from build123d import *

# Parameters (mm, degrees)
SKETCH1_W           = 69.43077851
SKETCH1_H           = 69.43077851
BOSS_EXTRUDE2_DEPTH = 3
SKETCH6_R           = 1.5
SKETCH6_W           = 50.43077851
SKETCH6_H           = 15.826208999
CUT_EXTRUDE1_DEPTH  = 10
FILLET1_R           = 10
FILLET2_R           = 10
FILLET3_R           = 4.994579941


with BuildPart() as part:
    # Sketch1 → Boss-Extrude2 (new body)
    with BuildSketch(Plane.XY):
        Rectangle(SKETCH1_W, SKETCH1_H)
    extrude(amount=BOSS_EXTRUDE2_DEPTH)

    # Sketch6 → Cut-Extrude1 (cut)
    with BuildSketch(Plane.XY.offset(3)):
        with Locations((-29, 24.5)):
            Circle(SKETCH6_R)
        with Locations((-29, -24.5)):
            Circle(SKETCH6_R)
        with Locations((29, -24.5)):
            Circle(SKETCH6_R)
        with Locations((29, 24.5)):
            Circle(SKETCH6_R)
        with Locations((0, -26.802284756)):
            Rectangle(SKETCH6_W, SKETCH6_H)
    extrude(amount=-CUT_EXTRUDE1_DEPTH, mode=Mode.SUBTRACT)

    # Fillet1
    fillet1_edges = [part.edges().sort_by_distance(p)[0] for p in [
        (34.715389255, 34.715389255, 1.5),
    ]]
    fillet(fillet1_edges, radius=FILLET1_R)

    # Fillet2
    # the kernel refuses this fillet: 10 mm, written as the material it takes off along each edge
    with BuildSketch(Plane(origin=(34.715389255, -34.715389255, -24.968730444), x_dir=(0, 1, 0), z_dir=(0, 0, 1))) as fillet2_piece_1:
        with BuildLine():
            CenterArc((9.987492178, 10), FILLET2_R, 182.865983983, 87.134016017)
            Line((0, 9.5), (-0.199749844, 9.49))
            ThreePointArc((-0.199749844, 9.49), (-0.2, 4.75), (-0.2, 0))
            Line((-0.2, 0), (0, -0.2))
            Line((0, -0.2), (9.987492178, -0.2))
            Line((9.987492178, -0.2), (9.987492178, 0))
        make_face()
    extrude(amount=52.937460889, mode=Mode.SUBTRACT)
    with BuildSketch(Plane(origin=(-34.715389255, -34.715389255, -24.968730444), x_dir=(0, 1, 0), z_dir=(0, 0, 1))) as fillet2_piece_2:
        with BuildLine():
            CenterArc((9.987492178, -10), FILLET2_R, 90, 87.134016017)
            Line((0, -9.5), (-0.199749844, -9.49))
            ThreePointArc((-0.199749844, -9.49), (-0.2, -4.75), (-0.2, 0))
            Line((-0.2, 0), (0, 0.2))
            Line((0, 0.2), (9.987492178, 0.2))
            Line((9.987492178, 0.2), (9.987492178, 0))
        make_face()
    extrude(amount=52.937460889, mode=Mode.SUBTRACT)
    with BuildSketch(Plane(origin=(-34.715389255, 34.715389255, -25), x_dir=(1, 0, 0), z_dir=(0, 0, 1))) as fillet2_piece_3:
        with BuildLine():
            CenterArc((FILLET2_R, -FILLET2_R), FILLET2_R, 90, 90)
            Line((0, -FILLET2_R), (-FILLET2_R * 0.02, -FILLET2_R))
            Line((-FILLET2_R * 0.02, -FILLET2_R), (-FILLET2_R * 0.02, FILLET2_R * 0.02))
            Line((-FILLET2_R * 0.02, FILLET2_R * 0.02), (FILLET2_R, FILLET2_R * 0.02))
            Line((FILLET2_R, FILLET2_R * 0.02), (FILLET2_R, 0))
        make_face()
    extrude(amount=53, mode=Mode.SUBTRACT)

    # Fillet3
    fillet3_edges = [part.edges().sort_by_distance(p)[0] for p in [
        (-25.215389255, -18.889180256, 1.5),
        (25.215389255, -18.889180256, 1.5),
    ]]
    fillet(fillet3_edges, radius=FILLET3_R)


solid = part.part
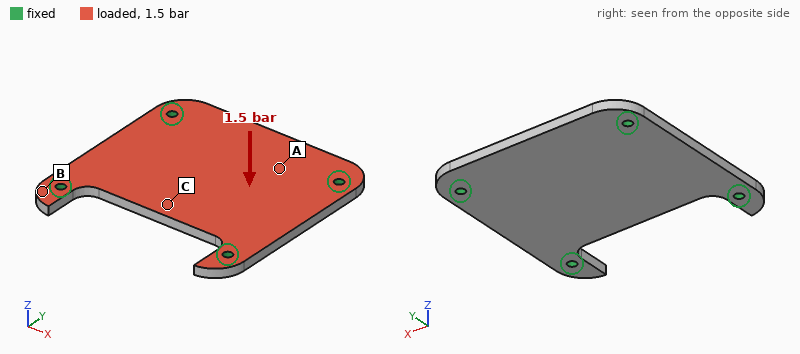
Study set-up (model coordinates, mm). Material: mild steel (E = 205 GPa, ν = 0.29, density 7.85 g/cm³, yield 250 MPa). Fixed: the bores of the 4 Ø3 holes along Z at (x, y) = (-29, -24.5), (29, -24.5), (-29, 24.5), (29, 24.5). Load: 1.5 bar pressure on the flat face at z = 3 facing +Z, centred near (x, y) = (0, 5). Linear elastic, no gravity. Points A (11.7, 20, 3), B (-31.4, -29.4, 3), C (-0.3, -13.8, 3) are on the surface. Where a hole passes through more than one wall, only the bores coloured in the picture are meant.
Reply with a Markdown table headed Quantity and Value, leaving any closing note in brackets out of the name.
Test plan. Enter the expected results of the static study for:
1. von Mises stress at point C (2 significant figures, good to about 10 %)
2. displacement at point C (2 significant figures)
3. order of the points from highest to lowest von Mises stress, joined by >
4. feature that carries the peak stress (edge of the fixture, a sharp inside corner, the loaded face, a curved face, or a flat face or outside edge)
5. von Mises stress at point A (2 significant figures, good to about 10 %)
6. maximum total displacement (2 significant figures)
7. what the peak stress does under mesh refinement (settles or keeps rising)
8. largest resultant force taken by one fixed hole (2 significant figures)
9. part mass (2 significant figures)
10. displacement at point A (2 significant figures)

| Quantity | Value |
|---|---|
| von Mises stress at point C | 19 MPa |
| displacement at point C | 21 µm |
| order of the points from highest to lowest von Mises stress, joined by > | C > A > B |
| feature that carries the peak stress | edge of the fixture |
| von Mises stress at point A | 12 MPa |
| maximum total displacement | 22 µm |
| what the peak stress does under mesh refinement | keeps rising |
| largest resultant force taken by one fixed hole | 180 N |
| part mass | 92 g |
| displacement at point A | 12 µm |
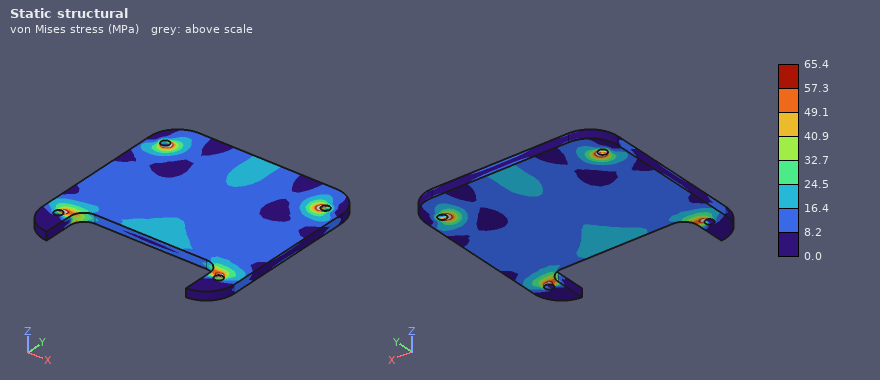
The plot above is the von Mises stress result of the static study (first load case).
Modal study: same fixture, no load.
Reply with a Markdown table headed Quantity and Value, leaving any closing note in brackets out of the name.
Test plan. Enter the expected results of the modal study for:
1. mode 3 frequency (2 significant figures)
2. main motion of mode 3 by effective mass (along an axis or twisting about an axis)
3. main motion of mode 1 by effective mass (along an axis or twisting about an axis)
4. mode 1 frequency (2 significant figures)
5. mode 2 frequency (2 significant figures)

| Quantity | Value |
|---|---|
| mode 3 frequency | 6400 Hz |
| main motion of mode 3 by effective mass | twisting about Y |
| main motion of mode 1 by effective mass | along Z |
| mode 1 frequency | 3200 Hz |
| mode 2 frequency | 5100 Hz |
